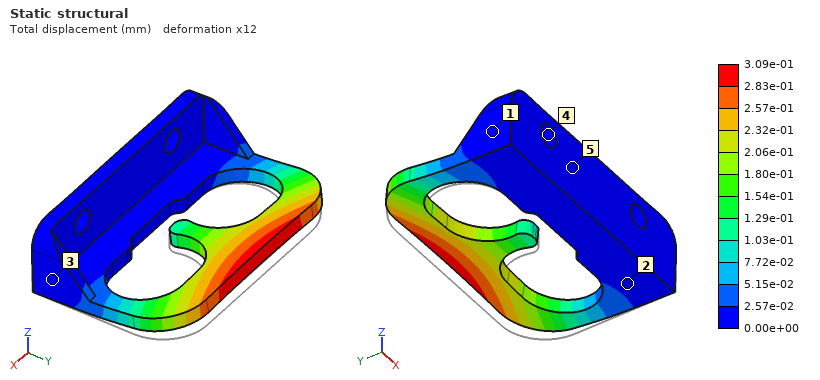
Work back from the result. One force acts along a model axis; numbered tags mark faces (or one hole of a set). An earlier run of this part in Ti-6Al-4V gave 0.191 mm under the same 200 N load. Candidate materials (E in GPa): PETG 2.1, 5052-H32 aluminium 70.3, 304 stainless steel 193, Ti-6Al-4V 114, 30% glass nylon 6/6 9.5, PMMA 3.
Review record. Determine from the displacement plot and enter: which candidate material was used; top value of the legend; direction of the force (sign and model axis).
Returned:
5052-H32 aluminium
3.09e-01 mm
+Z
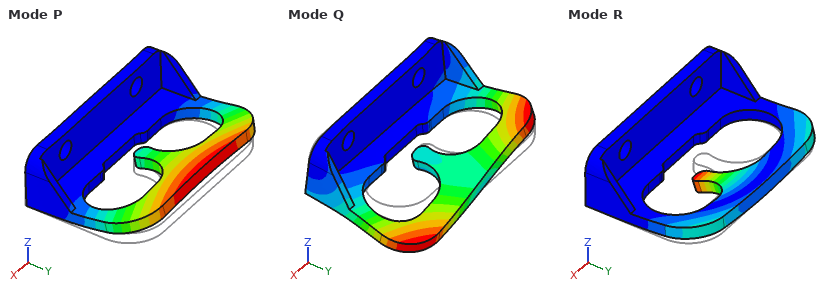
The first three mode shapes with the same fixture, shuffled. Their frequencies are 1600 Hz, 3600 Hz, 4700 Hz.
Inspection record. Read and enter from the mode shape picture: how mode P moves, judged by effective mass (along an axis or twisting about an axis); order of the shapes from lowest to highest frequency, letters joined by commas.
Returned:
along Z
P, Q, R
